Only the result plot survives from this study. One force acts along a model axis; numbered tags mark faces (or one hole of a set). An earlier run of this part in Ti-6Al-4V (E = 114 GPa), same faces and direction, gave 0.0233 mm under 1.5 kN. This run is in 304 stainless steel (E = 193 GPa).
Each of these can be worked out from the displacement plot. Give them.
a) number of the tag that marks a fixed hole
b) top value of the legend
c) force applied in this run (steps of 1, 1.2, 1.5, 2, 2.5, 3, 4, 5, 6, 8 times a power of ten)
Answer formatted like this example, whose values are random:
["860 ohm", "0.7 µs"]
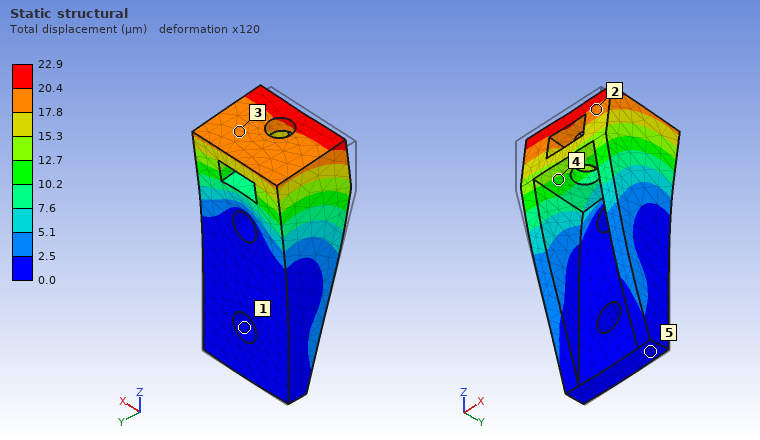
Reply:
["1", "22.9 µm", "2.5 kN"]
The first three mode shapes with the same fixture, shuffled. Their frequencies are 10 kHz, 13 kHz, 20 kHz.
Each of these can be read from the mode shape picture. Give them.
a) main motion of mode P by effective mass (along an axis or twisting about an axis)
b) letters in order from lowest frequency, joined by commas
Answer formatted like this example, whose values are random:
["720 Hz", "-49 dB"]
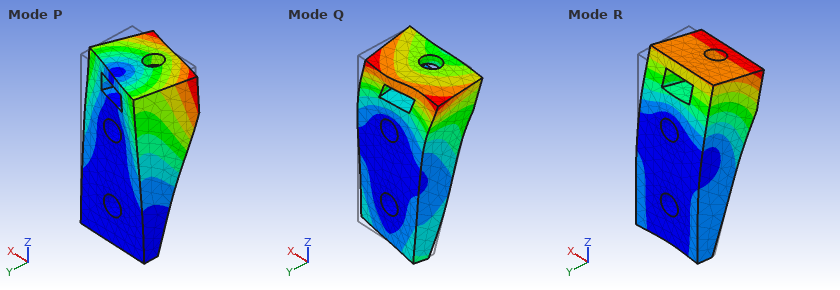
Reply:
["along X", "P, R, Q"]
